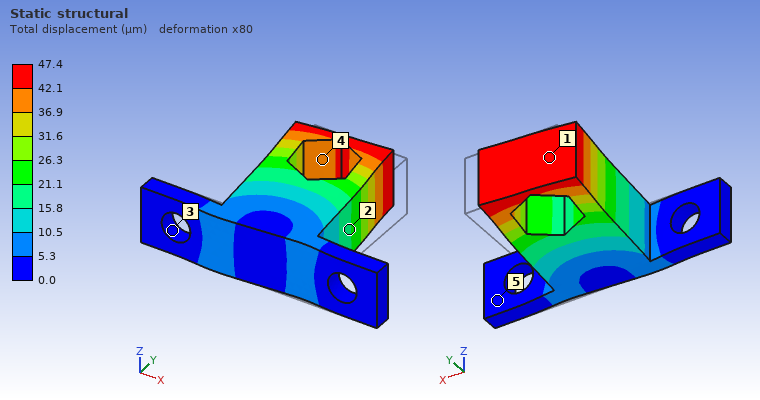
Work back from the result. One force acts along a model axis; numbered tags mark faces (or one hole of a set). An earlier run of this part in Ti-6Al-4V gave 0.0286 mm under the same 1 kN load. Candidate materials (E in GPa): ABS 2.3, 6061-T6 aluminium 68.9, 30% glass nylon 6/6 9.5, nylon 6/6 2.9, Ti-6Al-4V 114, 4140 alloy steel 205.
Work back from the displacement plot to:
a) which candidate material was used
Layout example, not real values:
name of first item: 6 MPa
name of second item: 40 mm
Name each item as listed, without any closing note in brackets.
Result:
which candidate material was used: 6061-T6 aluminium
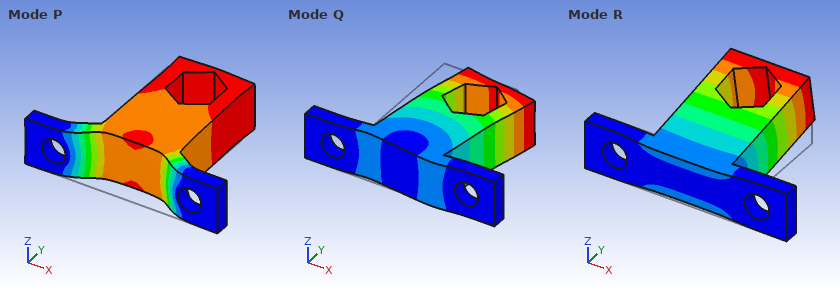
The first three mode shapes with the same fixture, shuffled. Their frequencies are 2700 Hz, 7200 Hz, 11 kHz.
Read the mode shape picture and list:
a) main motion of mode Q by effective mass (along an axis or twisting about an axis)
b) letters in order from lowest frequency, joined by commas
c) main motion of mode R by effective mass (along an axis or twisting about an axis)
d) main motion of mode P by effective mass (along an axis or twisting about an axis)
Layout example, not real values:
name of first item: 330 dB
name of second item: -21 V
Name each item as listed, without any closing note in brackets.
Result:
main motion of mode Q by effective mass: along X
letters in order from lowest frequency, joined by commas: R, Q, P
main motion of mode R by effective mass: along Z
main motion of mode P by effective mass: along Y
